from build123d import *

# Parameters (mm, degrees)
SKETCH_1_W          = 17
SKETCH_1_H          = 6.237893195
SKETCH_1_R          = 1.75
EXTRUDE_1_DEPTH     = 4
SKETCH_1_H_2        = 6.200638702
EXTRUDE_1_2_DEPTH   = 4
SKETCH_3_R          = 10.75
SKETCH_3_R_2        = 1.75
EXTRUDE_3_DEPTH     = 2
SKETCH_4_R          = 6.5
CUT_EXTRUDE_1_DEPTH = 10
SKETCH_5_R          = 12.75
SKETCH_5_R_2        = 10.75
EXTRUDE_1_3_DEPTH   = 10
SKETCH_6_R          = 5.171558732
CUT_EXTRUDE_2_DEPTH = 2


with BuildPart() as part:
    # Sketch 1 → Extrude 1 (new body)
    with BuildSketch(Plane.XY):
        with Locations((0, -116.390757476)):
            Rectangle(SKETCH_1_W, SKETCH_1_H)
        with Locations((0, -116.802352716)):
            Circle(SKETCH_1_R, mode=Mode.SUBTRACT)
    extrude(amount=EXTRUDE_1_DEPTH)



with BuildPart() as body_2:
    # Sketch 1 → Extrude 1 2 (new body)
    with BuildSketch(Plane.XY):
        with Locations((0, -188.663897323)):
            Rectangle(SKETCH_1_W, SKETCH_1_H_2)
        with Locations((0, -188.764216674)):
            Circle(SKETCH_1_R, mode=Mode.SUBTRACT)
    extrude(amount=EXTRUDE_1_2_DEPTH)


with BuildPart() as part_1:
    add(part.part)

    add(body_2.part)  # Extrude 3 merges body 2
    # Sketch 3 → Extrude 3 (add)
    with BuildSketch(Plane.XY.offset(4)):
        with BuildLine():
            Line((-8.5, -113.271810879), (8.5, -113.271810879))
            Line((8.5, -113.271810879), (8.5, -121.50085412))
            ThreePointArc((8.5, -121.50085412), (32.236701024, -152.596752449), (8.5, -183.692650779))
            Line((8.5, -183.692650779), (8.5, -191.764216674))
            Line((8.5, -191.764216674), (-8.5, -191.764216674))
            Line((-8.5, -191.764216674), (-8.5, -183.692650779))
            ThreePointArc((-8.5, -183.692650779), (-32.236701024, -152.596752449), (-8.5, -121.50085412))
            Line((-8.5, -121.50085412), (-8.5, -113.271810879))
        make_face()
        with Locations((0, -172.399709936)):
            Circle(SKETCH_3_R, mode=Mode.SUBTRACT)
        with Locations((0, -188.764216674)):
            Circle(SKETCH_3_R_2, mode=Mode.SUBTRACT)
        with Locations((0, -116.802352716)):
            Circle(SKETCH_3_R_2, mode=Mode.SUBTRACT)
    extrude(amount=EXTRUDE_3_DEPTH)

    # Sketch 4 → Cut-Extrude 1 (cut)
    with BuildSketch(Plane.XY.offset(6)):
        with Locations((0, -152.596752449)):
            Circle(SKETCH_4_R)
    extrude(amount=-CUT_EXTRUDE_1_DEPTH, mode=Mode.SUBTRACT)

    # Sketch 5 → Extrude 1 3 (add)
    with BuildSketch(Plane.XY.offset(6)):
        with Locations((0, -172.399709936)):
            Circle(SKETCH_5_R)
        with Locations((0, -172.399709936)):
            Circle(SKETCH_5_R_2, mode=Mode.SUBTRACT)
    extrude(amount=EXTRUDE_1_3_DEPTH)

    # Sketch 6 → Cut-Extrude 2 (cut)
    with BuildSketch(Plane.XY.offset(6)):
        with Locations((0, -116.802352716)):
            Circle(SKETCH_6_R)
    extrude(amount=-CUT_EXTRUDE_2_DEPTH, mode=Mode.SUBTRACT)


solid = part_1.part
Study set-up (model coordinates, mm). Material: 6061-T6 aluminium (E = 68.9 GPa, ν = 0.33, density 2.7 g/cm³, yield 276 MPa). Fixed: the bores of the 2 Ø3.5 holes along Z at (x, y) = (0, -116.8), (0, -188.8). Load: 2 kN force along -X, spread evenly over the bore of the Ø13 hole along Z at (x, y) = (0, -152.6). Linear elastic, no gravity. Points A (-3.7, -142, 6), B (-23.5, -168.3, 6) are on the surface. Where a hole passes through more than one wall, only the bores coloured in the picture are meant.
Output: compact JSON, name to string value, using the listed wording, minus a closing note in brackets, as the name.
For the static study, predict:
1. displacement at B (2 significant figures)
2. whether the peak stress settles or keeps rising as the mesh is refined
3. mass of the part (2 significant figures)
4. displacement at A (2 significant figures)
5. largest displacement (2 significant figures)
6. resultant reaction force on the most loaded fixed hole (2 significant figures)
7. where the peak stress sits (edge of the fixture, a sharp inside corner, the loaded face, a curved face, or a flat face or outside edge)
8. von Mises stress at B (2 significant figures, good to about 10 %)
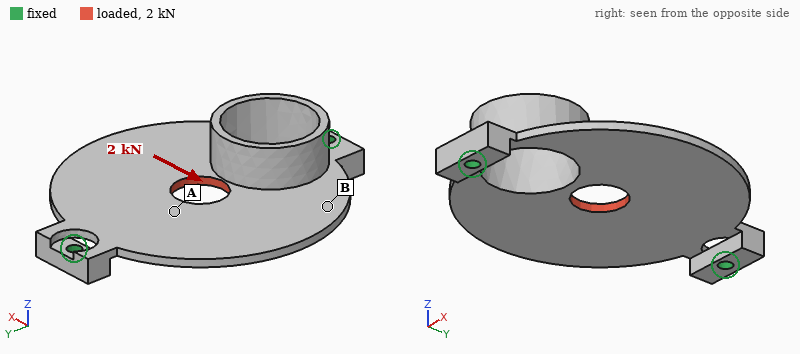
{"displacement at B": "31 µm", "whether the peak stress settles or keeps rising as the mesh is refined": "keeps rising", "mass of the part": "22 g", "displacement at A": "44 µm", "largest displacement": "47 µm", "resultant reaction force on the most loaded fixed hole": "1.0 kN", "where the peak stress sits": "a sharp inside corner", "von Mises stress at B": "34 MPa"}
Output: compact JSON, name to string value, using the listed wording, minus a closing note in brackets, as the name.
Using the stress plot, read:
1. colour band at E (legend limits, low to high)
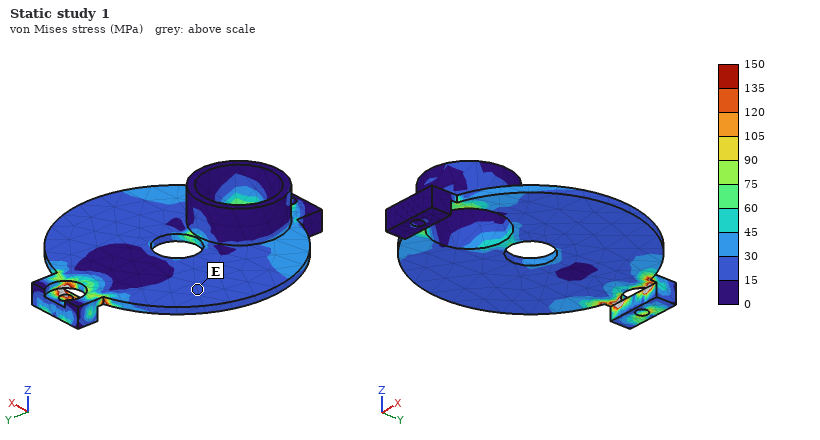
{"colour band at E": "15 to 30 MPa"}
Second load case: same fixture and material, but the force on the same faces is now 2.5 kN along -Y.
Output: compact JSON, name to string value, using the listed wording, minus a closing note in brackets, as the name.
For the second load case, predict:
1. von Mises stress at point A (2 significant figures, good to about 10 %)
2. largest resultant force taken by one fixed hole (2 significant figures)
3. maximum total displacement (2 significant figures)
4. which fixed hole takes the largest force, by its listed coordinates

{"von Mises stress at point A": "33 MPa", "largest resultant force taken by one fixed hole": "1.4 kN", "maximum total displacement": "73 µm", "which fixed hole takes the largest force, by its listed coordinates": "(0, -116.8)"}
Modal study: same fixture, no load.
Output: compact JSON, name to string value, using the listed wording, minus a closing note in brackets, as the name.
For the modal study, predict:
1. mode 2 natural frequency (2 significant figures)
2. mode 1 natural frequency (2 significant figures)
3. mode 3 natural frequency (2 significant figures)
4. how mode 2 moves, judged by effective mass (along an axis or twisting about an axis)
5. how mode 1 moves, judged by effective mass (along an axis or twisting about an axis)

{"mode 2 natural frequency": "1600 Hz", "mode 1 natural frequency": "1400 Hz", "mode 3 natural frequency": "3800 Hz", "how mode 2 moves, judged by effective mass": "twisting about Y", "how mode 1 moves, judged by effective mass": "along Z"}
